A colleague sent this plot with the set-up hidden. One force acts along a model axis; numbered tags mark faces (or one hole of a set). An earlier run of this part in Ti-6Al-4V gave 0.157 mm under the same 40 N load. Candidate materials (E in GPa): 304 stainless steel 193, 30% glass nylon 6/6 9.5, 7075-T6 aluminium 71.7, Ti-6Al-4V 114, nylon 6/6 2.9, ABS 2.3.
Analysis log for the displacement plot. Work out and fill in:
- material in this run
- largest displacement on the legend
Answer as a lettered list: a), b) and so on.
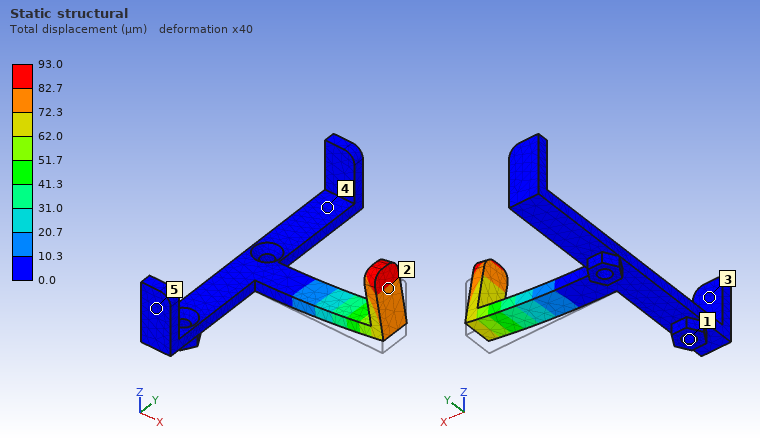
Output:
a) 304 stainless steel
b) 93.0 µm
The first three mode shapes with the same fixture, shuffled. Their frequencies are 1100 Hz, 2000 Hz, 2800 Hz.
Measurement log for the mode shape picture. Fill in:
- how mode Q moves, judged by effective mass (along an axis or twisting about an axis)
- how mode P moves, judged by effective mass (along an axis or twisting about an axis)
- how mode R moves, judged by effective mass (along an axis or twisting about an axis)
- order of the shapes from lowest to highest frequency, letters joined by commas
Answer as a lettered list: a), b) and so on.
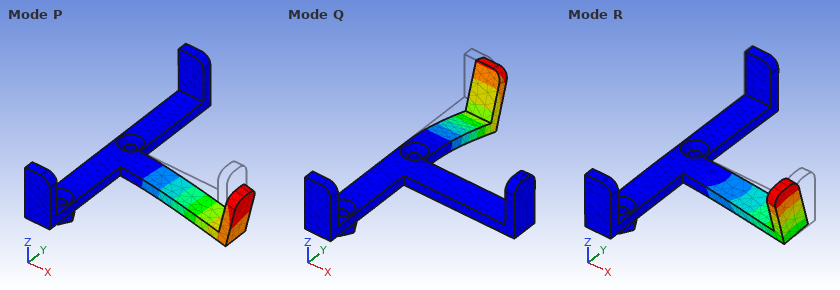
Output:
a) along Z
b) along Z
c) along Y
d) P, Q, R
